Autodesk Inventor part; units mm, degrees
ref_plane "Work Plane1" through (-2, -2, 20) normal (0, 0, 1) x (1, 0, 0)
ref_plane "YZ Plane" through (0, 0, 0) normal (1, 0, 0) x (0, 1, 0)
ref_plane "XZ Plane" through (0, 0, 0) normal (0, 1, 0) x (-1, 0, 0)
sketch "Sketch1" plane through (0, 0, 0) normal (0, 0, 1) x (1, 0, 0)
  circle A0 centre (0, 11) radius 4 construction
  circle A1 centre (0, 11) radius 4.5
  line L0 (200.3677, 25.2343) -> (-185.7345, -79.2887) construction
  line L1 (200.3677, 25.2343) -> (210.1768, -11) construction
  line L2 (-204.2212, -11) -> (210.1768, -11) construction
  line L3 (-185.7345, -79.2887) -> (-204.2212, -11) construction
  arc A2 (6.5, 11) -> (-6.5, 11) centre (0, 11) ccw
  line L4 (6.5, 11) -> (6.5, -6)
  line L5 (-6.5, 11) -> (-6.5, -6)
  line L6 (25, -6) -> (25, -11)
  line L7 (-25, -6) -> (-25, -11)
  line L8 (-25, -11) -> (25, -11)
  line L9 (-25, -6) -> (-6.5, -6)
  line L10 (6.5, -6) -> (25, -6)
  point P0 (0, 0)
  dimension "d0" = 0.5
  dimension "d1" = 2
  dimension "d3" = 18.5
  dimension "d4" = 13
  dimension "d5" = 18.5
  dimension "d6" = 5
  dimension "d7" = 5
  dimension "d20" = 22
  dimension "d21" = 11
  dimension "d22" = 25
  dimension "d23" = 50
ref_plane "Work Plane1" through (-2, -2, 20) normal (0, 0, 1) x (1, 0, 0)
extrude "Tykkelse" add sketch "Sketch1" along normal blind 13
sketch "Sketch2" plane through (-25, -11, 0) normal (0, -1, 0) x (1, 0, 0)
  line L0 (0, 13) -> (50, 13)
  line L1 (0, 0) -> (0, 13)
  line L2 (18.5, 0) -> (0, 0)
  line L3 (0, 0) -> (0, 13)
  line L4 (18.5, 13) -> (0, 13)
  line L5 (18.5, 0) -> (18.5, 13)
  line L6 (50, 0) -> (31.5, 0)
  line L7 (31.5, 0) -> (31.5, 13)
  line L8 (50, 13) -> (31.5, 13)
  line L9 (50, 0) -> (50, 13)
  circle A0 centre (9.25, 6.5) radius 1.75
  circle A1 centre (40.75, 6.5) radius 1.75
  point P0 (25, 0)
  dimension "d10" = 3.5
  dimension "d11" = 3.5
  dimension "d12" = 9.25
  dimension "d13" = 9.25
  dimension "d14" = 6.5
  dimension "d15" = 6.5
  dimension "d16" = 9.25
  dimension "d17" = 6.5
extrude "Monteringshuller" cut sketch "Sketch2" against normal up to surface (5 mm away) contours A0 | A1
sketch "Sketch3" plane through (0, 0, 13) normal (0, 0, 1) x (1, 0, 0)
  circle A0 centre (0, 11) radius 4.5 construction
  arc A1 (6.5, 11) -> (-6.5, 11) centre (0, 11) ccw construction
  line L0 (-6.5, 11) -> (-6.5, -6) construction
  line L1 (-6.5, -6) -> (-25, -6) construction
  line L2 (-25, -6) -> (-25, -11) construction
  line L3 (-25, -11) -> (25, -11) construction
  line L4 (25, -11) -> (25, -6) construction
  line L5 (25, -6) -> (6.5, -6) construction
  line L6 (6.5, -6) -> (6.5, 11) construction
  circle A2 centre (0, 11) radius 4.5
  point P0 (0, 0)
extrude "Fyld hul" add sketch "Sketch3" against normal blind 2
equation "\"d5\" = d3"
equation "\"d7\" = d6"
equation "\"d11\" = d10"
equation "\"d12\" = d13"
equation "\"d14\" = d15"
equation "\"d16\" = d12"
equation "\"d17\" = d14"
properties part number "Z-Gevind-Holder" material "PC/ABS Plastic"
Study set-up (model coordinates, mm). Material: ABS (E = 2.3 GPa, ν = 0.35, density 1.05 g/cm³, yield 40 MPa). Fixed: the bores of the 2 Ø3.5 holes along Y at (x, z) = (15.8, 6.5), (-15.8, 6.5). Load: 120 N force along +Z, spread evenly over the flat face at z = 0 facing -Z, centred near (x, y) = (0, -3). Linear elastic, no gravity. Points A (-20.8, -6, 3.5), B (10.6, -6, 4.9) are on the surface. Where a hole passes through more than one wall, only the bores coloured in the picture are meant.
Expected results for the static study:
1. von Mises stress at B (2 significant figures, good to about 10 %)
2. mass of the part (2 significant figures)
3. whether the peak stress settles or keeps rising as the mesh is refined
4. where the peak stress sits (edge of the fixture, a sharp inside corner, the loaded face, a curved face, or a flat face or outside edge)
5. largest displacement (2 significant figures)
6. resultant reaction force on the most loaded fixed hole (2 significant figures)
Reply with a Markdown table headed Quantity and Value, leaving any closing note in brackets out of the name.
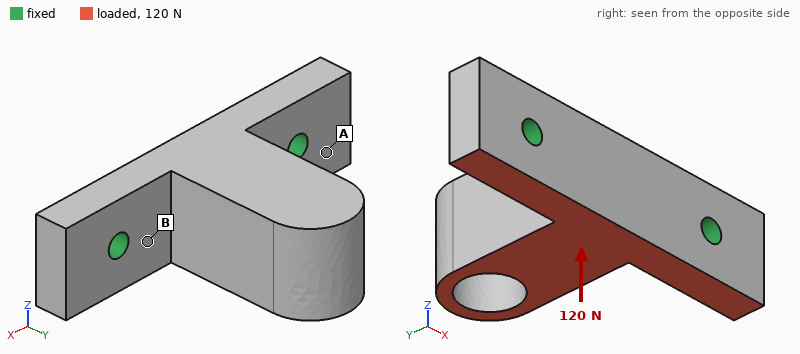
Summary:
| Quantity | Value |
|---|---|
| von Mises stress at B | 6.5 MPa |
| mass of the part | 6.5 g |
| whether the peak stress settles or keeps rising as the mesh is refined | keeps rising |
| where the peak stress sits | edge of the fixture |
| largest displacement | 0.27 mm |
| resultant reaction force on the most loaded fixed hole | 60 N |
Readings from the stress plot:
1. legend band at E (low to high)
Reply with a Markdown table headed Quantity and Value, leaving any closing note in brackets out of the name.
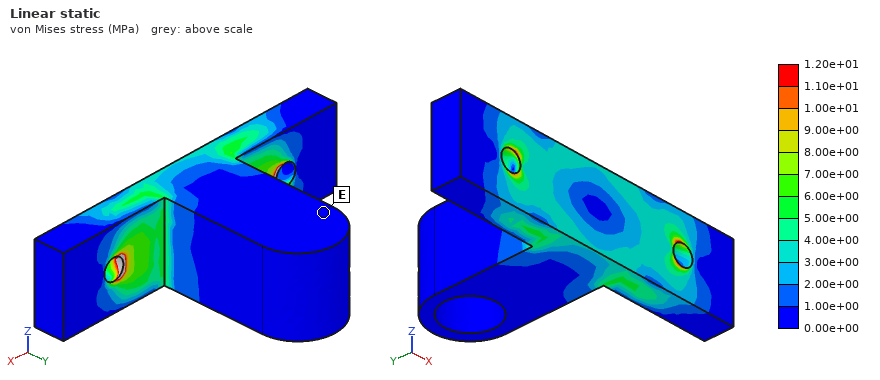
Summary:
| Quantity | Value |
|---|---|
| legend band at E | 0.00e+00 to 1.00e+00 MPa |
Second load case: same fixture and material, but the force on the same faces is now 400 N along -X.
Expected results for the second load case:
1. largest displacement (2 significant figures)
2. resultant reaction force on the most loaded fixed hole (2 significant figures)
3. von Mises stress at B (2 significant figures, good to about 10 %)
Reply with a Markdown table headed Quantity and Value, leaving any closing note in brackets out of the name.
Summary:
| Quantity | Value |
|---|---|
| largest displacement | 0.27 mm |
| resultant reaction force on the most loaded fixed hole | 230 N |
| von Mises stress at B | 6.4 MPa |
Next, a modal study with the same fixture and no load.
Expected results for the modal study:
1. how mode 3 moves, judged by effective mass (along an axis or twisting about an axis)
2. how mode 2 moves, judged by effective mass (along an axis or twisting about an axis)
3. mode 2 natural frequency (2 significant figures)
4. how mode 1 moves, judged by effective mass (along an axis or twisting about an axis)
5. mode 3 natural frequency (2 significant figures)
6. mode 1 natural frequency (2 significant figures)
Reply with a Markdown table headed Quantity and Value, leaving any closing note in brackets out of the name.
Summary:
| Quantity | Value |
|---|---|
| how mode 3 moves, judged by effective mass | along Y |
| how mode 2 moves, judged by effective mass | along X |
| mode 2 natural frequency | 3200 Hz |
| how mode 1 moves, judged by effective mass | along Z |
| mode 3 natural frequency | 4300 Hz |
| mode 1 natural frequency | 1600 Hz |
